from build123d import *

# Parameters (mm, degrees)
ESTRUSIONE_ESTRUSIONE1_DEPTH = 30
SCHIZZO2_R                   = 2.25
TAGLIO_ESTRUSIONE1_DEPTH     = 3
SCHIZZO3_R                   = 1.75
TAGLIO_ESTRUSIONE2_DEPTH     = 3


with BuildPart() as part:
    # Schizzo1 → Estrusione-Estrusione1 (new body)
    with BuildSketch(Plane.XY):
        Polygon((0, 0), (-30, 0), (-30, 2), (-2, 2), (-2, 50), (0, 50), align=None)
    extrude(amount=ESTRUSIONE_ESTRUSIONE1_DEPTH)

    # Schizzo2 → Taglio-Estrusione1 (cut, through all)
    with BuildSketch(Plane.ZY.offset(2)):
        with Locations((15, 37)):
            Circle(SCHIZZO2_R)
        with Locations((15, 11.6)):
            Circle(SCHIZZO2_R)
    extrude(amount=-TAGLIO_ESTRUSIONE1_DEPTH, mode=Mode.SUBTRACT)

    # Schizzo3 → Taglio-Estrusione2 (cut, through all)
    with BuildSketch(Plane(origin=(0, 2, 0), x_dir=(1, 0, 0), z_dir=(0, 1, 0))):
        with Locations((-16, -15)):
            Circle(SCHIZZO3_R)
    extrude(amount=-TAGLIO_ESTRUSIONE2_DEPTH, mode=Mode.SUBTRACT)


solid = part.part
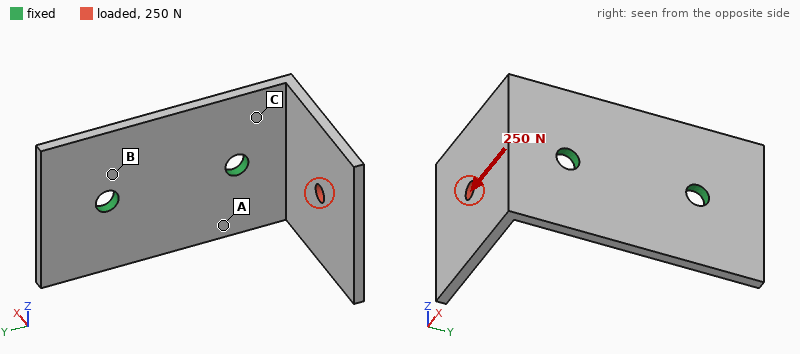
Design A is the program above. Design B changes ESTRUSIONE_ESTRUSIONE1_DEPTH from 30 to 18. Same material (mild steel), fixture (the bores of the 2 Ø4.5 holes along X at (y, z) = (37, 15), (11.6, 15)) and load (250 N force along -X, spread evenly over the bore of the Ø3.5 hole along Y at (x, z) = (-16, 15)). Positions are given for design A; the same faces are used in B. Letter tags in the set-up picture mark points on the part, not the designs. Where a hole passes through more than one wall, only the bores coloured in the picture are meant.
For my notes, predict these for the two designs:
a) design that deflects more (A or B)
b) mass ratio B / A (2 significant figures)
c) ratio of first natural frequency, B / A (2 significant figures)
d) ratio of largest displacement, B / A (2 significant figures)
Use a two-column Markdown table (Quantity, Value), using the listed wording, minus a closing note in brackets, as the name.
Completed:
| Quantity | Value |
|---|---|
| design that deflects more | B |
| mass ratio B / A | 0.59 |
| ratio of first natural frequency, B / A | 0.99 |
| ratio of largest displacement, B / A | 1.6 |
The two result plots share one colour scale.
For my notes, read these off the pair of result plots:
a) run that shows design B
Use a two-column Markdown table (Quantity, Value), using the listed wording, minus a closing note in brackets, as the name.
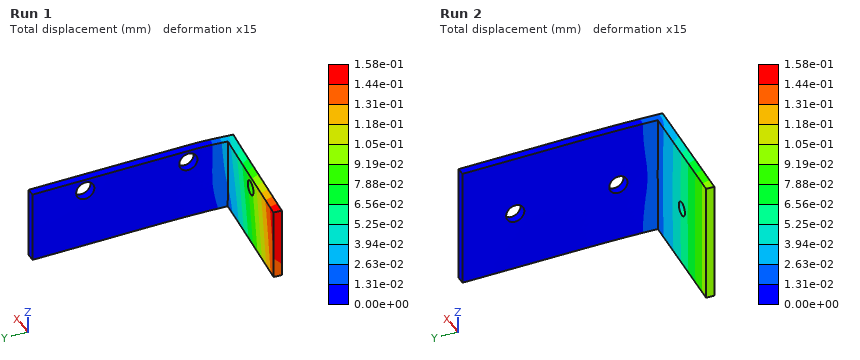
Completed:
| Quantity | Value |
|---|---|
| run that shows design B | Run 1 |
